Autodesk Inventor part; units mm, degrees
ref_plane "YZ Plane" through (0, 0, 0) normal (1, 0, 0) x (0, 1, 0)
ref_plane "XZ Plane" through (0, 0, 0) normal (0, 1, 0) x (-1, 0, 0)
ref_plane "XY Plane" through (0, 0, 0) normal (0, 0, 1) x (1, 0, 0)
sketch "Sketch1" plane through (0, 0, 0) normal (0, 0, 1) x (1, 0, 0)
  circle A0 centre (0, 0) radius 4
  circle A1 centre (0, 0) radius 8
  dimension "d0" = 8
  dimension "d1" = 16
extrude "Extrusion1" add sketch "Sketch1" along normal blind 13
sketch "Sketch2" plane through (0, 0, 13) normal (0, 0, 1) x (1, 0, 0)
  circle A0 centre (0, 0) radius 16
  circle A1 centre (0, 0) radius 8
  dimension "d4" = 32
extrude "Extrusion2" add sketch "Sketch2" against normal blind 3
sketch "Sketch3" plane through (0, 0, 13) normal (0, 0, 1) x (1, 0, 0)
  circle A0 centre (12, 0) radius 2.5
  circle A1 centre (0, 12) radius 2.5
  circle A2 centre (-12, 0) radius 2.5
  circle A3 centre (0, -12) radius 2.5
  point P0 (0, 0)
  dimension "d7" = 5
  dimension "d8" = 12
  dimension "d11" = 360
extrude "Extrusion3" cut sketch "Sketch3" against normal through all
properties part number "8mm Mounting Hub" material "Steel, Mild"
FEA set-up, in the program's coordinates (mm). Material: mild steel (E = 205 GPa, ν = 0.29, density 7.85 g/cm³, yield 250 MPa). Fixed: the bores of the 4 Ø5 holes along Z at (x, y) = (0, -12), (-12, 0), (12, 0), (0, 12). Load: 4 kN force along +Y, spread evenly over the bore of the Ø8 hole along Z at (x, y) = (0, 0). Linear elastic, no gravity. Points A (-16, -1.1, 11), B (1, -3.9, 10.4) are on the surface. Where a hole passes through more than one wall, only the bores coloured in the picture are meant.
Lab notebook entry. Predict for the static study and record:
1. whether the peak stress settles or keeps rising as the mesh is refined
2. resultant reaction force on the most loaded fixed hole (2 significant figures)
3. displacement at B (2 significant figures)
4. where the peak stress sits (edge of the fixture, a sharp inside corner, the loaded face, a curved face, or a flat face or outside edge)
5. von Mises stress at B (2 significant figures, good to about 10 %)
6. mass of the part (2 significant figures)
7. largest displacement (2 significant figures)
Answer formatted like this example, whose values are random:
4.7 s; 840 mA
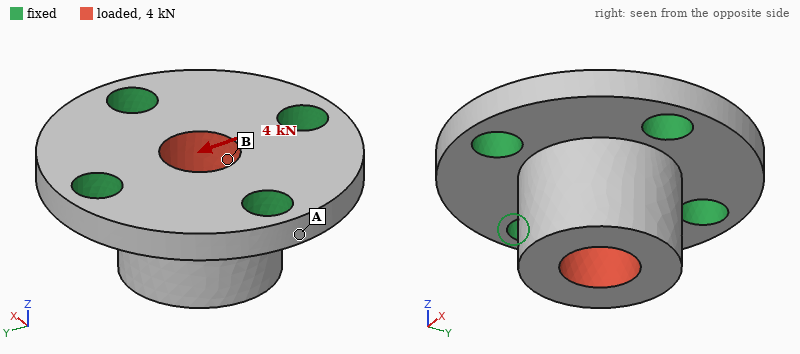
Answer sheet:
keeps rising; 1.6 kN; 1.5 µm; edge of the fixture; 34 MPa; 28 g; 7.3 µm
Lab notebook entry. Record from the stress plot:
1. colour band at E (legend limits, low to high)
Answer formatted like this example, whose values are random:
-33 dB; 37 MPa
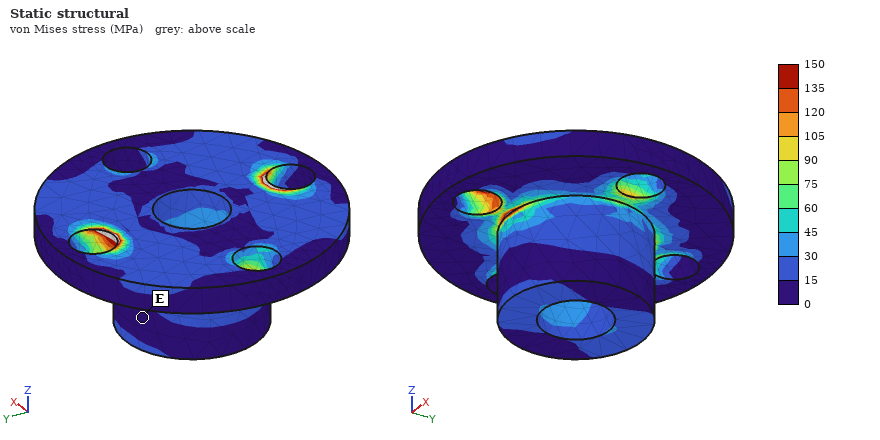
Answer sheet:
0 to 15 MPa
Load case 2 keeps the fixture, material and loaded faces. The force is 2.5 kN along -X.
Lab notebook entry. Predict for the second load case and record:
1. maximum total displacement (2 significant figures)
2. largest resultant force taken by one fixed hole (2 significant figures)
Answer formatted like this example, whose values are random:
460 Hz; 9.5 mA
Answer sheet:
4.6 µm; 1.0 kN
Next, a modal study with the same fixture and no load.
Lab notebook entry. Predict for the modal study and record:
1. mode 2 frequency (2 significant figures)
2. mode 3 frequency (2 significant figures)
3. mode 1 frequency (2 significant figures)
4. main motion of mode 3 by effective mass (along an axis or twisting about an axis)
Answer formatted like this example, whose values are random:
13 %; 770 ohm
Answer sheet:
34 kHz; 44 kHz; 34 kHz; along Z
